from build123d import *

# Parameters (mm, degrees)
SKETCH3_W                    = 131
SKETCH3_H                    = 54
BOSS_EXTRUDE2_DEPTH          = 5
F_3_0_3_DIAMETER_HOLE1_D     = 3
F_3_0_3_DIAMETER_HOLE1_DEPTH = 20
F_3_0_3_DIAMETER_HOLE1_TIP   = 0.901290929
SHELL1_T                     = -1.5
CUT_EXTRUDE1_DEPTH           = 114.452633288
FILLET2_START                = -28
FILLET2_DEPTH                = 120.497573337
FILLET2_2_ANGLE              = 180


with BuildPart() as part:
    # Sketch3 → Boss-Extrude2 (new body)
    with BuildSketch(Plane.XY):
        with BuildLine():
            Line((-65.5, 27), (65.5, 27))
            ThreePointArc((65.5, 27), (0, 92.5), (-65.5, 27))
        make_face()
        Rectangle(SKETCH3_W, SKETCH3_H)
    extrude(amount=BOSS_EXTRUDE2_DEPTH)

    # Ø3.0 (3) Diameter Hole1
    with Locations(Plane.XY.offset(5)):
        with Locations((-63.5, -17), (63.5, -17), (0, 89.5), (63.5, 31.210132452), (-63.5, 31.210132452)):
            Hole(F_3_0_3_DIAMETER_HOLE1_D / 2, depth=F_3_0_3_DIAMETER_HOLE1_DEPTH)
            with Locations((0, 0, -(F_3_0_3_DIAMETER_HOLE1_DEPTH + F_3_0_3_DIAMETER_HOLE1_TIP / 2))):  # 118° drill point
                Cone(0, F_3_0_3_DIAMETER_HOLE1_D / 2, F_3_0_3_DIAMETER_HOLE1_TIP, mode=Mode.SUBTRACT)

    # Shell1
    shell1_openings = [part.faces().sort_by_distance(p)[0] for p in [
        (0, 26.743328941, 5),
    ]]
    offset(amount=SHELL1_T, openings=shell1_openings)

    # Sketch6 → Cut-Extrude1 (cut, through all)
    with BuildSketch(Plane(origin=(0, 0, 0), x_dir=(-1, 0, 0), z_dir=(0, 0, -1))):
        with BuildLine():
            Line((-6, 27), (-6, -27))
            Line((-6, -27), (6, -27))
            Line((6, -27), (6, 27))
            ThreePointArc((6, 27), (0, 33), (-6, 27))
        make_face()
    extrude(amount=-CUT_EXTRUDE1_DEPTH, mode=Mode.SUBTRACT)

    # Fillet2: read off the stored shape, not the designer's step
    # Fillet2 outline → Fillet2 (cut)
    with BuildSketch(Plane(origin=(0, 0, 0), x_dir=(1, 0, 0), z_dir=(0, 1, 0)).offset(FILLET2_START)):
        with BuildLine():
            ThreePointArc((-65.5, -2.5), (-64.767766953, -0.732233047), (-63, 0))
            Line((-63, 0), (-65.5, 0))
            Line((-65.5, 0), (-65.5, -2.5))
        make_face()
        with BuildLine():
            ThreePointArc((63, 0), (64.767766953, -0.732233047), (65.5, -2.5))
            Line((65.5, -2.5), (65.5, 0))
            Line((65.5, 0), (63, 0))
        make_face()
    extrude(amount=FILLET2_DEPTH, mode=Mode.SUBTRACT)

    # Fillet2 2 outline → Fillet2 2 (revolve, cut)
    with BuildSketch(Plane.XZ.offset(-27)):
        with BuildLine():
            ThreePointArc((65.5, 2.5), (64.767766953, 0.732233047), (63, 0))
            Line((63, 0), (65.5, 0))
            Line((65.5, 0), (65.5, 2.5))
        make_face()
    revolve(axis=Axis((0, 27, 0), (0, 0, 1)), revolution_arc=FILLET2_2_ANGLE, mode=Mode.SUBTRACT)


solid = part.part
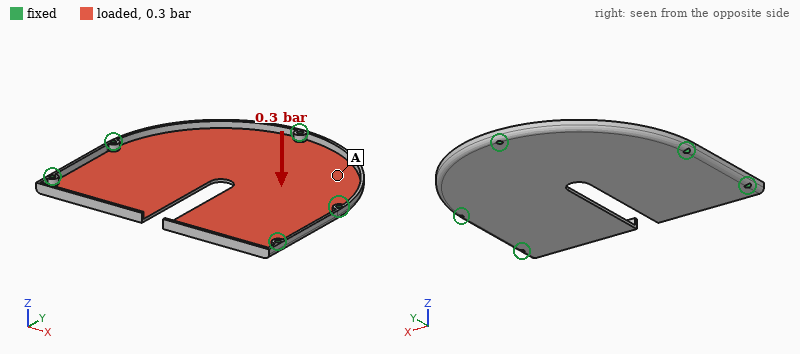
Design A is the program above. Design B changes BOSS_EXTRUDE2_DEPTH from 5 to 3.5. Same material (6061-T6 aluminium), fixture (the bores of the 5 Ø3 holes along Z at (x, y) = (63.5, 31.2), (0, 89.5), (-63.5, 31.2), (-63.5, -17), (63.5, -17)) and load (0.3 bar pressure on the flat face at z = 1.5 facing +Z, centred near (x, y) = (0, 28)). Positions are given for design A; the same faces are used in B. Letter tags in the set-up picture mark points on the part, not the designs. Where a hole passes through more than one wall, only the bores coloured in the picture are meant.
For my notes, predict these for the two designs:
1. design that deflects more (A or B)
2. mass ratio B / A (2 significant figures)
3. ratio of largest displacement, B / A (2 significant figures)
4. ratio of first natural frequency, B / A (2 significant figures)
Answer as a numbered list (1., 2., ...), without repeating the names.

1. B
2. 0.95
3. 1.3
4. 0.90
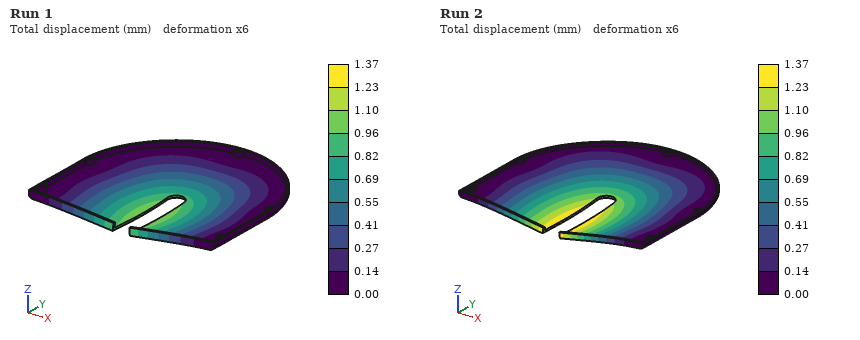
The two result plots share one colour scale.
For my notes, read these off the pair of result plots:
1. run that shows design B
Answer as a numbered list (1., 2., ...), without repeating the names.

1. Run 2
